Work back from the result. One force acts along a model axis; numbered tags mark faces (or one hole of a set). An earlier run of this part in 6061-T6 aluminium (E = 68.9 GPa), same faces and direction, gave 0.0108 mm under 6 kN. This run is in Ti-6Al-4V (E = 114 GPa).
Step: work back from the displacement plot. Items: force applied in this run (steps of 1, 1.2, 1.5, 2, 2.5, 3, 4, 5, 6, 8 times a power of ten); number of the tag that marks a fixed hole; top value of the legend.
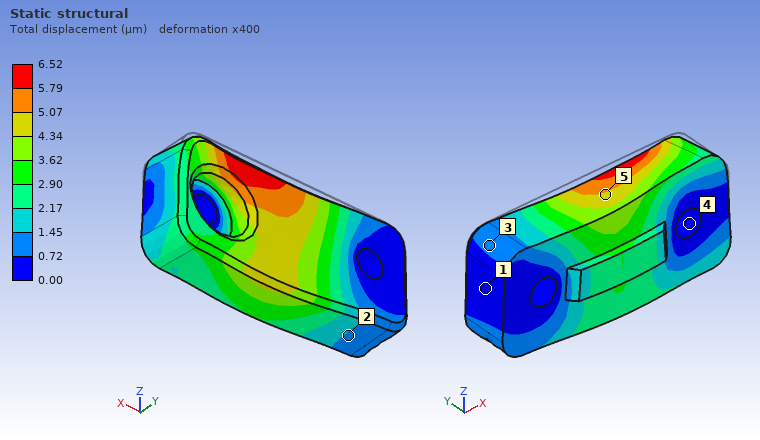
6 kN
4
6.52 µm
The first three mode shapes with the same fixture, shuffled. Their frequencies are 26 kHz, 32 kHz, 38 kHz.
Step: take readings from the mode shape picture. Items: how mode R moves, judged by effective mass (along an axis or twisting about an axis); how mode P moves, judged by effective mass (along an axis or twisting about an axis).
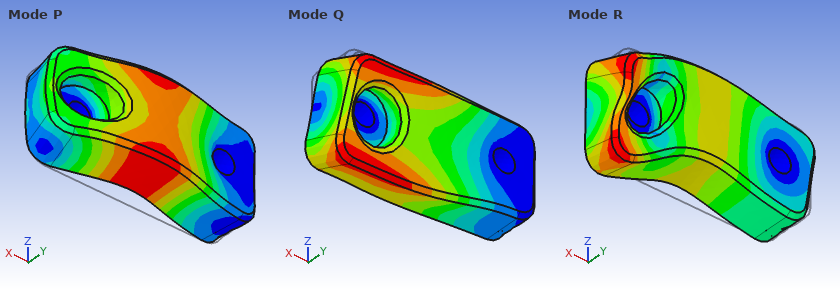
along Z
along Y
